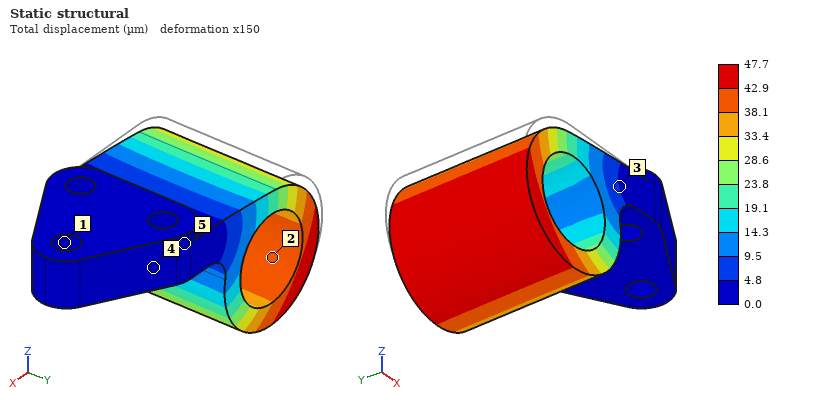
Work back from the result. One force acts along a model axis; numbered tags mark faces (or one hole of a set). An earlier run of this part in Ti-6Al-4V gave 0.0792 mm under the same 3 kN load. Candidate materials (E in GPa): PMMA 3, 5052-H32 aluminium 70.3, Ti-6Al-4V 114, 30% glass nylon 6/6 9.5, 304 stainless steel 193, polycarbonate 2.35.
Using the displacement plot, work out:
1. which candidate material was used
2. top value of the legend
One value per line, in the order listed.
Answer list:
304 stainless steel
47.7 µm
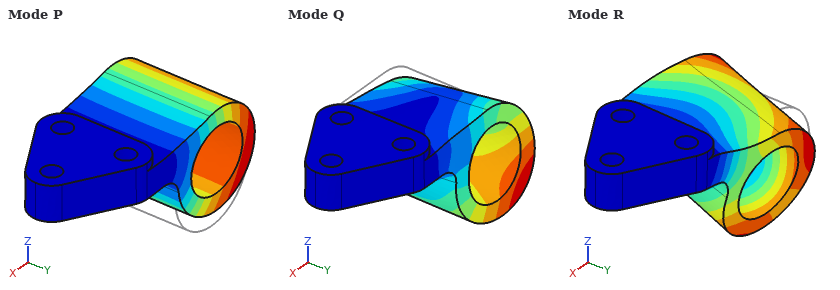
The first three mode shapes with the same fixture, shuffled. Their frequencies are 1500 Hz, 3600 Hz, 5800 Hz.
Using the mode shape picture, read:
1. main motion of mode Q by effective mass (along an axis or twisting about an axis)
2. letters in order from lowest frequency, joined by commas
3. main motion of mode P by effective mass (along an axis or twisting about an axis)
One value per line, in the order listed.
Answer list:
along Y
P, Q, R
along Z
